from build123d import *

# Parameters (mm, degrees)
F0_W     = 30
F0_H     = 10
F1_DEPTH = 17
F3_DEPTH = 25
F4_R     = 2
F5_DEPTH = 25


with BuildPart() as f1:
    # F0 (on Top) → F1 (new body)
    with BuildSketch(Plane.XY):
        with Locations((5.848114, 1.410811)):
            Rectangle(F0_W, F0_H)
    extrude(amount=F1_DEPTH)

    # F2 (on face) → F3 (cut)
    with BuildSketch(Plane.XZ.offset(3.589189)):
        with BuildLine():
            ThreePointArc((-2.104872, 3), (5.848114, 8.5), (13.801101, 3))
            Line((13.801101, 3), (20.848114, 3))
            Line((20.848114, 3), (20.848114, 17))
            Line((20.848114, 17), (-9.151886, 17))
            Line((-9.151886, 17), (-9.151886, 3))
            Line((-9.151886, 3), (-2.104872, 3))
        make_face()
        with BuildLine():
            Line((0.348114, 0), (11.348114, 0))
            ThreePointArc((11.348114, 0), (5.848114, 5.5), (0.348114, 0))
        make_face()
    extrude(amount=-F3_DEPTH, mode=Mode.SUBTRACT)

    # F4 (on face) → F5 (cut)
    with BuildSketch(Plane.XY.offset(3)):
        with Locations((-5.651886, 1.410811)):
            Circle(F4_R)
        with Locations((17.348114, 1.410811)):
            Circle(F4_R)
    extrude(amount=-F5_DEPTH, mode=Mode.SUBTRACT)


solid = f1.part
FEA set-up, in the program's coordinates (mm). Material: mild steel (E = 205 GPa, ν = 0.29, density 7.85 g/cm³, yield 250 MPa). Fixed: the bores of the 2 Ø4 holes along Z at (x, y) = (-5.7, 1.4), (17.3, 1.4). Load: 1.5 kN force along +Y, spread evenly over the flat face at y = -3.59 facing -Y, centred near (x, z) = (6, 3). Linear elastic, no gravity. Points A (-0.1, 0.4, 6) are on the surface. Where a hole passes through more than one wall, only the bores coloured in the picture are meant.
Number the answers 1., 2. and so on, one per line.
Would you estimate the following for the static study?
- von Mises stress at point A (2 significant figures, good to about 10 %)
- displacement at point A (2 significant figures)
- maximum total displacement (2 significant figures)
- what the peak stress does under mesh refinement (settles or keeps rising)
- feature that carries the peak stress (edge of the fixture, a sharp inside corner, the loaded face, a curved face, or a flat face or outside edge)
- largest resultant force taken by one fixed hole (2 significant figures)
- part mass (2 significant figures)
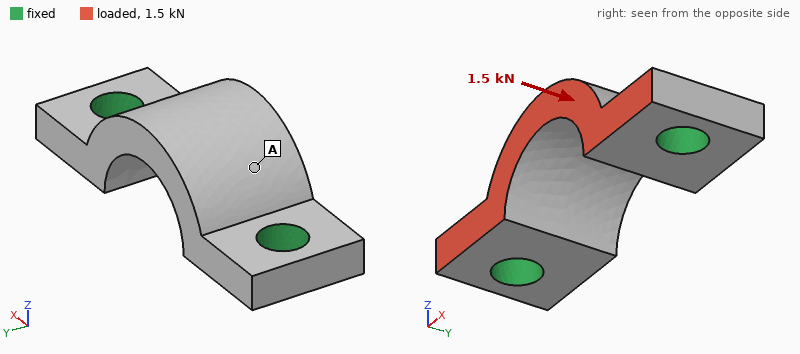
1. 37 MPa
2. 5.1 µm
3. 9.0 µm
4. keeps rising
5. edge of the fixture
6. 750 N
7. 7.7 g
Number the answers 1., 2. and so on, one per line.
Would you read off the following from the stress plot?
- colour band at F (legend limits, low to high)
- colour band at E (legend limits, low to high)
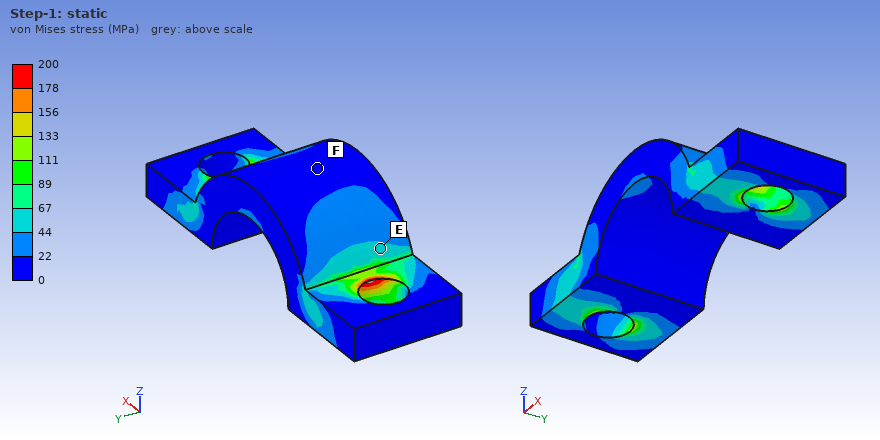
1. 0 to 22 MPa
2. 44 to 67 MPa
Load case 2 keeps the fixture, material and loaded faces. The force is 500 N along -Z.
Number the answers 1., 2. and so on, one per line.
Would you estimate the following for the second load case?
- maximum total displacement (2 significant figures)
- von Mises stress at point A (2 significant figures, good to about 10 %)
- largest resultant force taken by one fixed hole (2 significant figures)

1. 4.7 µm
2. 14 MPa
3. 270 N
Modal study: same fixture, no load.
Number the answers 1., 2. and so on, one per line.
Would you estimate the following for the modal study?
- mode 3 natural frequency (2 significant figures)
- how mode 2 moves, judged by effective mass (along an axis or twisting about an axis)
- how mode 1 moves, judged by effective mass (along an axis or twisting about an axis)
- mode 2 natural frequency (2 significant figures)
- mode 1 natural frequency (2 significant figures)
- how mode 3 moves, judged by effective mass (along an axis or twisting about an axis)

1. 55 kHz
2. along Z
3. along Y
4. 49 kHz
5. 27 kHz
6. along X
